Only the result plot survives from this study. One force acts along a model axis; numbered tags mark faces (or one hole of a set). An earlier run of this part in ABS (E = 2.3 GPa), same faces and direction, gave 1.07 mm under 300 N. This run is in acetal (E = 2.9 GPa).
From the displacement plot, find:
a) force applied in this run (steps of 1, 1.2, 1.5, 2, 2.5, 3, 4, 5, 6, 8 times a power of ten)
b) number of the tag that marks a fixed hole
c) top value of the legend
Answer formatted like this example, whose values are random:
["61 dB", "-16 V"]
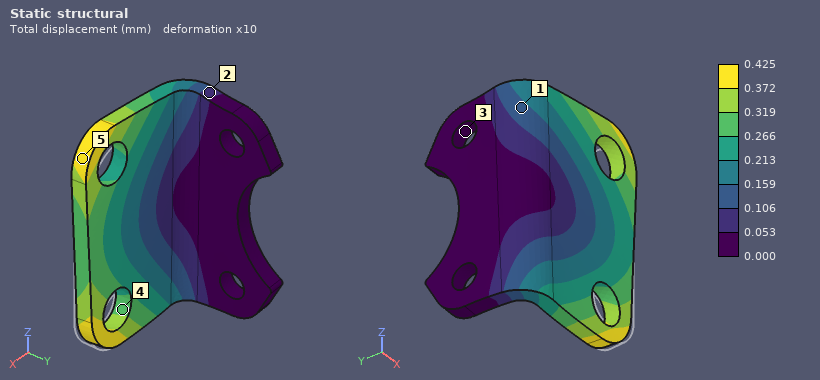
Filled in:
["150 N", "3", "0.425 mm"]
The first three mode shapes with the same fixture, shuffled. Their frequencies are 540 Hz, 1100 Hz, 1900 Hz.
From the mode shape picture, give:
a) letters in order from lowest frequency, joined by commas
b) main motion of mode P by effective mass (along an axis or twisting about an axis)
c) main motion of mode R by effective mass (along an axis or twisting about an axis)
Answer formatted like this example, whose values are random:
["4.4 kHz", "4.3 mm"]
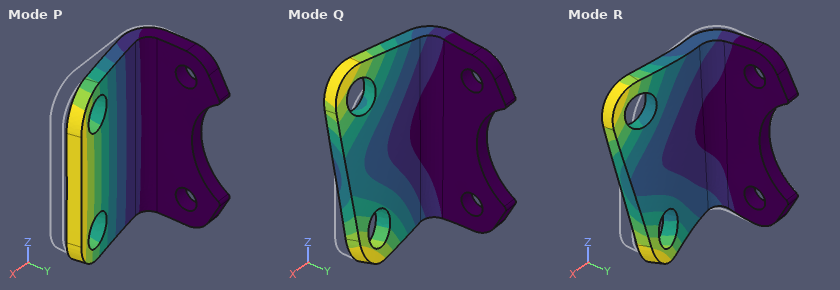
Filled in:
["P, Q, R", "along Y", "along Z"]
